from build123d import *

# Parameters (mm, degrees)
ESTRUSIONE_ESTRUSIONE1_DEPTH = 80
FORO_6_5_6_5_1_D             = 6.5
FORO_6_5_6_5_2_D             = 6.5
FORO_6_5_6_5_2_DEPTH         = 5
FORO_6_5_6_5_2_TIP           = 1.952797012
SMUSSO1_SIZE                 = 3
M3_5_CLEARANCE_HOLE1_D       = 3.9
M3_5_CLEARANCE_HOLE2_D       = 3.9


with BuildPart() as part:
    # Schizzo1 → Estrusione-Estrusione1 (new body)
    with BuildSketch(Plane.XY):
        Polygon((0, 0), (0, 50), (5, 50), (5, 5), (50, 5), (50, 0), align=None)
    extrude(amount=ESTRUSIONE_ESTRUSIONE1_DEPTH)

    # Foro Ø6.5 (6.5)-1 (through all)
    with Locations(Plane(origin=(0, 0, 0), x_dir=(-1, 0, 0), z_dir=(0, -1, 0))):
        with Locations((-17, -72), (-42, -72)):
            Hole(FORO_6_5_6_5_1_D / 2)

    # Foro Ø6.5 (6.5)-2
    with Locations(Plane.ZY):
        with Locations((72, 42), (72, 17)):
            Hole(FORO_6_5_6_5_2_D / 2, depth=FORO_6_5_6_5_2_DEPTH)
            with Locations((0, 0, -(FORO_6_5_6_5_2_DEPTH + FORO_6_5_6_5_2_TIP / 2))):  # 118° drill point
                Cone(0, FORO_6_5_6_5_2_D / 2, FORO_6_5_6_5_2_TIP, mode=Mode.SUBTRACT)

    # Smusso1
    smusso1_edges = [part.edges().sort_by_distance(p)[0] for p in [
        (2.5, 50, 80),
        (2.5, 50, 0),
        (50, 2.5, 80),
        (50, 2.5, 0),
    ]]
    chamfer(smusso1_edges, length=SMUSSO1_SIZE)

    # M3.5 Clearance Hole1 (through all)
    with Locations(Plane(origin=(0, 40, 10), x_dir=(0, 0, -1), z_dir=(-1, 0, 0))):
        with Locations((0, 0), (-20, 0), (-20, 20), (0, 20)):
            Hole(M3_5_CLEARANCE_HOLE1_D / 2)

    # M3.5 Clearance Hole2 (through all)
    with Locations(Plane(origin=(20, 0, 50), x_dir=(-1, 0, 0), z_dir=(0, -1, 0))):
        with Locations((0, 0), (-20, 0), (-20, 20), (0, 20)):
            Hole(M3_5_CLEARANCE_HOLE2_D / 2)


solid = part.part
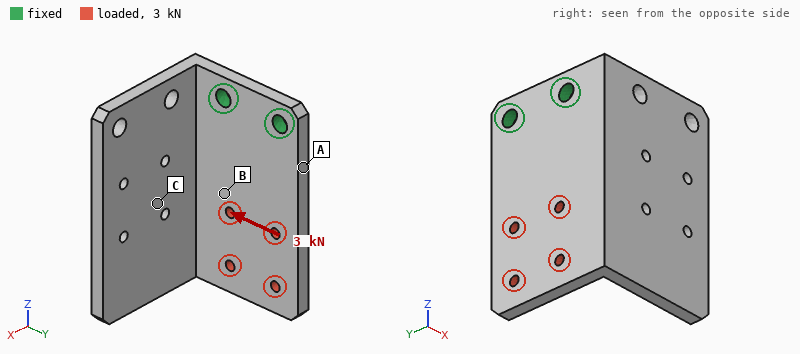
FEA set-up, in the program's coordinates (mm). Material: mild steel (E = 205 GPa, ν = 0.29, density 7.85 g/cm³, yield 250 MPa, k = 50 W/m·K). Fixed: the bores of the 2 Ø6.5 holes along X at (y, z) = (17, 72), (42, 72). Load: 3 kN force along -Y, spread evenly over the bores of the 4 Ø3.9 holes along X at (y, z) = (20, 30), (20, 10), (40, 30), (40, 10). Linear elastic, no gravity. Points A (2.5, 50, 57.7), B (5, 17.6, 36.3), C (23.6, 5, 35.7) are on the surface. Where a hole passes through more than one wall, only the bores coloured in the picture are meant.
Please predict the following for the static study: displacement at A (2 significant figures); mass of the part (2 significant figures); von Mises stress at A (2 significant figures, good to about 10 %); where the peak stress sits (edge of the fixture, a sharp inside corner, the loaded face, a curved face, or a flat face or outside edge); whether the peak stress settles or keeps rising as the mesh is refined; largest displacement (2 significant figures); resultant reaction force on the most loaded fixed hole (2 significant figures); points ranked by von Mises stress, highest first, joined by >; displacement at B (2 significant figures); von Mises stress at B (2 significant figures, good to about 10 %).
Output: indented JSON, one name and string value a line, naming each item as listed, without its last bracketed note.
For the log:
{
  "displacement at A": "9.2 µm",
  "mass of the part": "290 g",
  "von Mises stress at A": "58 MPa",
  "where the peak stress sits": "edge of the fixture",
  "whether the peak stress settles or keeps rising as the mesh is refined": "keeps rising",
  "largest displacement": "42 µm",
  "resultant reaction force on the most loaded fixed hole": "5.4 kN",
  "points ranked by von Mises stress, highest first, joined by >": "A > B > C",
  "displacement at B": "19 µm",
  "von Mises stress at B": "26 MPa"
}
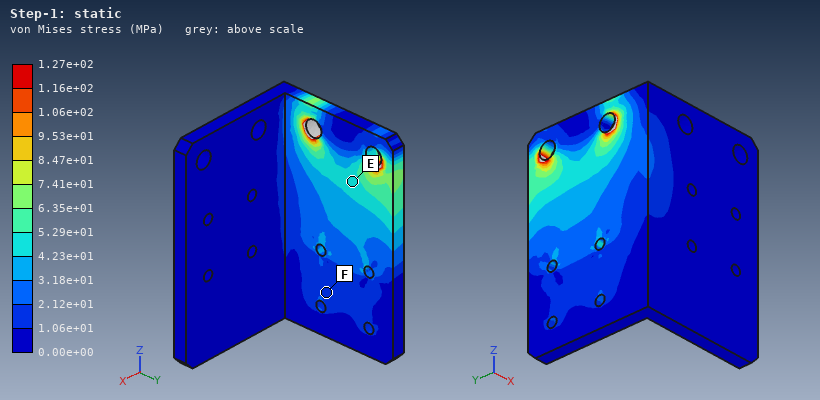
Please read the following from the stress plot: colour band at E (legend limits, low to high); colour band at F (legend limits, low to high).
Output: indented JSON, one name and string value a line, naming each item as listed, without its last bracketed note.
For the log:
{
  "colour band at E": "4.23e+01 to 5.29e+01 MPa",
  "colour band at F": "1.06e+01 to 2.12e+01 MPa"
}
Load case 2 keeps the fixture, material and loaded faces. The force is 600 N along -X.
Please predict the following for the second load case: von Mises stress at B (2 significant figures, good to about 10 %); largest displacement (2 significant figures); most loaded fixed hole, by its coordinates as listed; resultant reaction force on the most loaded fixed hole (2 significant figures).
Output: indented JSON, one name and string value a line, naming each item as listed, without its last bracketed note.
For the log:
{
  "von Mises stress at B": "28 MPa",
  "largest displacement": "0.22 mm",
  "most loaded fixed hole, by its coordinates as listed": "(17, 72)",
  "resultant reaction force on the most loaded fixed hole": "370 N"
}
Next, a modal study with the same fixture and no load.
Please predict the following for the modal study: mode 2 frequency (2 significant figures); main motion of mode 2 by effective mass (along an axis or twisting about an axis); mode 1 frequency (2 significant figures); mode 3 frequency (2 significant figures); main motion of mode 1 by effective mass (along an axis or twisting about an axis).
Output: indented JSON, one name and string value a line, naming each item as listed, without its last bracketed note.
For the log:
{
  "mode 2 frequency": "1000 Hz",
  "main motion of mode 2 by effective mass": "along Y",
  "mode 1 frequency": "690 Hz",
  "mode 3 frequency": "2300 Hz",
  "main motion of mode 1 by effective mass": "along X"
}
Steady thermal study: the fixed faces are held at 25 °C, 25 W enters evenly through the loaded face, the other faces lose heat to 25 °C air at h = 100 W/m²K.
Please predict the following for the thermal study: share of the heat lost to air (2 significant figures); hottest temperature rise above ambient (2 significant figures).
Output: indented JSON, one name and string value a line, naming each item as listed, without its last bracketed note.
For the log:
{
  "share of the heat lost to air": "77 %",
  "hottest temperature rise above ambient": "40 K"
}
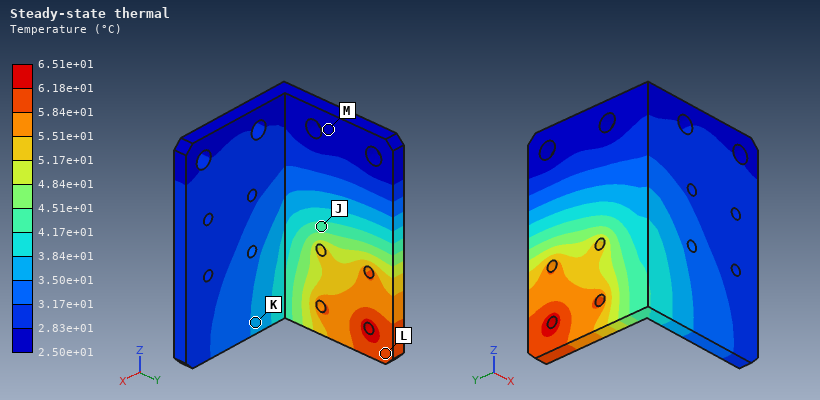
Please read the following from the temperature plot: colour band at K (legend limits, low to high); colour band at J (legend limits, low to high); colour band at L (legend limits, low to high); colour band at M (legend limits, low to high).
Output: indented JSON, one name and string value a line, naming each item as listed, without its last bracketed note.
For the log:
{
  "colour band at K": "3.50e+01 to 3.84e+01 °C",
  "colour band at J": "4.17e+01 to 4.51e+01 °C",
  "colour band at L": "5.84e+01 to 6.18e+01 °C",
  "colour band at M": "2.50e+01 to 2.83e+01 °C"
}
